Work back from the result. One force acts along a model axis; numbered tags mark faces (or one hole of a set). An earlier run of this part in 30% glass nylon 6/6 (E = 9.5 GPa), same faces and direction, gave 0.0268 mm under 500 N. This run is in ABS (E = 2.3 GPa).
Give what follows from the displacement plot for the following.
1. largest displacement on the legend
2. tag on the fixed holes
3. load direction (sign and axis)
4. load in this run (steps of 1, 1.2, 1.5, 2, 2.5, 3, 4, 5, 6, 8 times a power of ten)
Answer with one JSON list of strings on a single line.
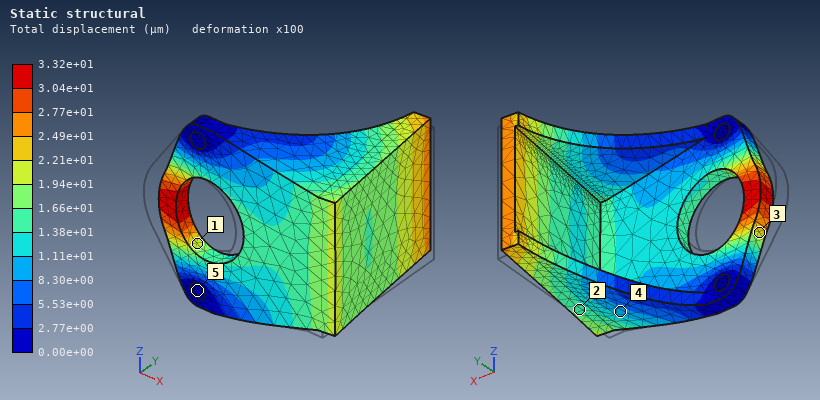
["3.32e+01 µm", "5", "+X", "150 N"]
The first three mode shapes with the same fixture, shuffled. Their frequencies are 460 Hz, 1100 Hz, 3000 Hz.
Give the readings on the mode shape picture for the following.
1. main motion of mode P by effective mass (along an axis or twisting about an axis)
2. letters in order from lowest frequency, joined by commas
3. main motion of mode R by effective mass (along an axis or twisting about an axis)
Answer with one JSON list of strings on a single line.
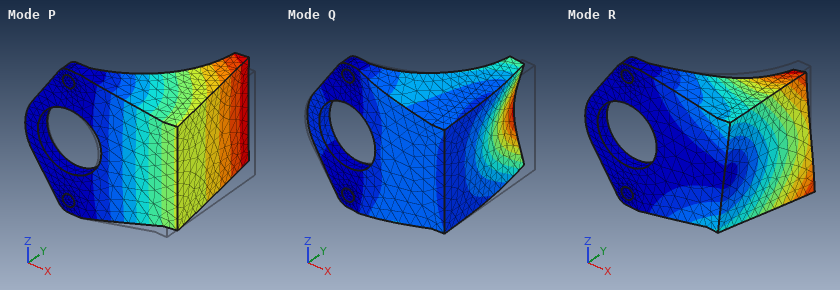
["along Y", "P, R, Q", "along Z"]
